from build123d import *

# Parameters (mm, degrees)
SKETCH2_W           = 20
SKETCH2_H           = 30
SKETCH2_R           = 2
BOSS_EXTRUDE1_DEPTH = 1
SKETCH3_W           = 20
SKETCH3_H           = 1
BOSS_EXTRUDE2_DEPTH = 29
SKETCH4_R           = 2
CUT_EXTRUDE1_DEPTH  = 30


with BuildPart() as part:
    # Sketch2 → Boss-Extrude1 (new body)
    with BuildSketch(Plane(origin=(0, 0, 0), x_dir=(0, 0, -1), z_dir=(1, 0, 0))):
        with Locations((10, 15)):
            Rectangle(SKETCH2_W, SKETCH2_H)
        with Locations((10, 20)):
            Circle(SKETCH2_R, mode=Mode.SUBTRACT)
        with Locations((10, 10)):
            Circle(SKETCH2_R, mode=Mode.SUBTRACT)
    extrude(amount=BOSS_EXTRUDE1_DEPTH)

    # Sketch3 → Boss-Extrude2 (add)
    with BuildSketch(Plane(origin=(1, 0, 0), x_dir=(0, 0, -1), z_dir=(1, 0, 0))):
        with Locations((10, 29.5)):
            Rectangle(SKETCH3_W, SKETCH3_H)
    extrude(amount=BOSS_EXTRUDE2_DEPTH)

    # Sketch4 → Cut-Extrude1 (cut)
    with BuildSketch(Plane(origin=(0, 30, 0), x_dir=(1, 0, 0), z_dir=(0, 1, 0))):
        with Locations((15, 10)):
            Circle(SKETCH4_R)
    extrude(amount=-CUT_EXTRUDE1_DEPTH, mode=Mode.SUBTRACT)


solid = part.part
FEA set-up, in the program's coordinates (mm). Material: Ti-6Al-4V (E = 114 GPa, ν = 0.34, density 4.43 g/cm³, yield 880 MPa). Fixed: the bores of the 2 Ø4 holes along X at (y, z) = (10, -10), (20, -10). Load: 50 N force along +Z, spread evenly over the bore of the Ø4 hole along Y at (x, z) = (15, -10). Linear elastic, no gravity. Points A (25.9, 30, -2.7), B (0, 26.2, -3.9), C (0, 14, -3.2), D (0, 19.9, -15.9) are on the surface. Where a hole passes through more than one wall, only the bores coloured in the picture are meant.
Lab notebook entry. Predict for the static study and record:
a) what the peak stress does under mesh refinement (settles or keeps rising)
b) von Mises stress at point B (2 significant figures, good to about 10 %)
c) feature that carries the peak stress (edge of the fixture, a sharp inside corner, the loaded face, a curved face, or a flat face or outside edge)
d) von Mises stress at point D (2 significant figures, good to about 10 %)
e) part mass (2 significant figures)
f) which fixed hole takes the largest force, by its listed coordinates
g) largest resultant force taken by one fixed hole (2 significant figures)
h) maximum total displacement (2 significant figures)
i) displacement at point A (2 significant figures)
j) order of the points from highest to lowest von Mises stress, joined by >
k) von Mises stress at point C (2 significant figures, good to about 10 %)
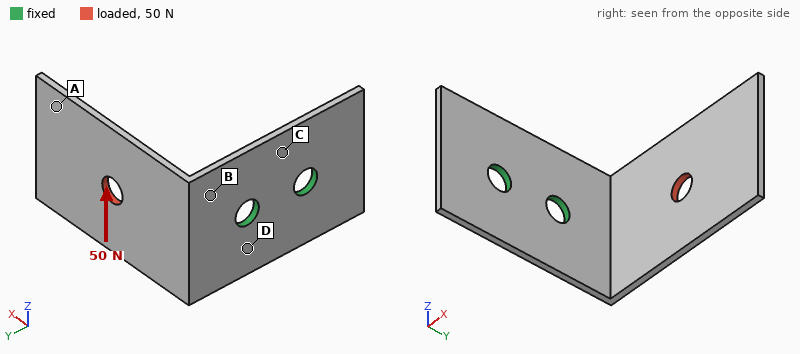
keeps rising
70 MPa
edge of the fixture
110 MPa
5.1 g
(20, -10)
77 N
0.49 mm
0.41 mm
D > B > C > A
43 MPa
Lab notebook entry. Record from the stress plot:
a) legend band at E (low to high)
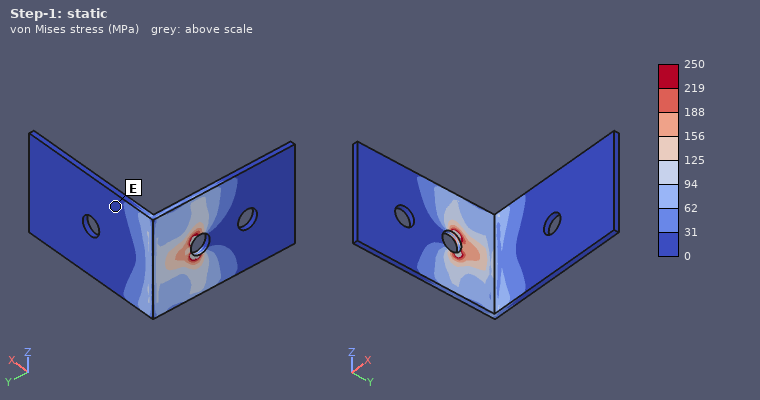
0 to 31 MPa
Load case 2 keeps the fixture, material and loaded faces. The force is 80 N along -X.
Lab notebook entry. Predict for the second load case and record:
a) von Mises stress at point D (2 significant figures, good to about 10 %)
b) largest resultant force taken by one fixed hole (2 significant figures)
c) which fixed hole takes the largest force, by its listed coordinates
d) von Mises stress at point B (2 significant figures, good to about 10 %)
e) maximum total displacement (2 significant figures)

69 MPa
93 N
(20, -10)
71 MPa
0.47 mm
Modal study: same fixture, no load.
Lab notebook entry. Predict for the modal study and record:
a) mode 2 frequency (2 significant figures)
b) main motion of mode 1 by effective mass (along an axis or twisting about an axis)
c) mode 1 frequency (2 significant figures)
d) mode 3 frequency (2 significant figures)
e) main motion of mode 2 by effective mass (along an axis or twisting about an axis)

1200 Hz
along Y
660 Hz
2900 Hz
along Z
